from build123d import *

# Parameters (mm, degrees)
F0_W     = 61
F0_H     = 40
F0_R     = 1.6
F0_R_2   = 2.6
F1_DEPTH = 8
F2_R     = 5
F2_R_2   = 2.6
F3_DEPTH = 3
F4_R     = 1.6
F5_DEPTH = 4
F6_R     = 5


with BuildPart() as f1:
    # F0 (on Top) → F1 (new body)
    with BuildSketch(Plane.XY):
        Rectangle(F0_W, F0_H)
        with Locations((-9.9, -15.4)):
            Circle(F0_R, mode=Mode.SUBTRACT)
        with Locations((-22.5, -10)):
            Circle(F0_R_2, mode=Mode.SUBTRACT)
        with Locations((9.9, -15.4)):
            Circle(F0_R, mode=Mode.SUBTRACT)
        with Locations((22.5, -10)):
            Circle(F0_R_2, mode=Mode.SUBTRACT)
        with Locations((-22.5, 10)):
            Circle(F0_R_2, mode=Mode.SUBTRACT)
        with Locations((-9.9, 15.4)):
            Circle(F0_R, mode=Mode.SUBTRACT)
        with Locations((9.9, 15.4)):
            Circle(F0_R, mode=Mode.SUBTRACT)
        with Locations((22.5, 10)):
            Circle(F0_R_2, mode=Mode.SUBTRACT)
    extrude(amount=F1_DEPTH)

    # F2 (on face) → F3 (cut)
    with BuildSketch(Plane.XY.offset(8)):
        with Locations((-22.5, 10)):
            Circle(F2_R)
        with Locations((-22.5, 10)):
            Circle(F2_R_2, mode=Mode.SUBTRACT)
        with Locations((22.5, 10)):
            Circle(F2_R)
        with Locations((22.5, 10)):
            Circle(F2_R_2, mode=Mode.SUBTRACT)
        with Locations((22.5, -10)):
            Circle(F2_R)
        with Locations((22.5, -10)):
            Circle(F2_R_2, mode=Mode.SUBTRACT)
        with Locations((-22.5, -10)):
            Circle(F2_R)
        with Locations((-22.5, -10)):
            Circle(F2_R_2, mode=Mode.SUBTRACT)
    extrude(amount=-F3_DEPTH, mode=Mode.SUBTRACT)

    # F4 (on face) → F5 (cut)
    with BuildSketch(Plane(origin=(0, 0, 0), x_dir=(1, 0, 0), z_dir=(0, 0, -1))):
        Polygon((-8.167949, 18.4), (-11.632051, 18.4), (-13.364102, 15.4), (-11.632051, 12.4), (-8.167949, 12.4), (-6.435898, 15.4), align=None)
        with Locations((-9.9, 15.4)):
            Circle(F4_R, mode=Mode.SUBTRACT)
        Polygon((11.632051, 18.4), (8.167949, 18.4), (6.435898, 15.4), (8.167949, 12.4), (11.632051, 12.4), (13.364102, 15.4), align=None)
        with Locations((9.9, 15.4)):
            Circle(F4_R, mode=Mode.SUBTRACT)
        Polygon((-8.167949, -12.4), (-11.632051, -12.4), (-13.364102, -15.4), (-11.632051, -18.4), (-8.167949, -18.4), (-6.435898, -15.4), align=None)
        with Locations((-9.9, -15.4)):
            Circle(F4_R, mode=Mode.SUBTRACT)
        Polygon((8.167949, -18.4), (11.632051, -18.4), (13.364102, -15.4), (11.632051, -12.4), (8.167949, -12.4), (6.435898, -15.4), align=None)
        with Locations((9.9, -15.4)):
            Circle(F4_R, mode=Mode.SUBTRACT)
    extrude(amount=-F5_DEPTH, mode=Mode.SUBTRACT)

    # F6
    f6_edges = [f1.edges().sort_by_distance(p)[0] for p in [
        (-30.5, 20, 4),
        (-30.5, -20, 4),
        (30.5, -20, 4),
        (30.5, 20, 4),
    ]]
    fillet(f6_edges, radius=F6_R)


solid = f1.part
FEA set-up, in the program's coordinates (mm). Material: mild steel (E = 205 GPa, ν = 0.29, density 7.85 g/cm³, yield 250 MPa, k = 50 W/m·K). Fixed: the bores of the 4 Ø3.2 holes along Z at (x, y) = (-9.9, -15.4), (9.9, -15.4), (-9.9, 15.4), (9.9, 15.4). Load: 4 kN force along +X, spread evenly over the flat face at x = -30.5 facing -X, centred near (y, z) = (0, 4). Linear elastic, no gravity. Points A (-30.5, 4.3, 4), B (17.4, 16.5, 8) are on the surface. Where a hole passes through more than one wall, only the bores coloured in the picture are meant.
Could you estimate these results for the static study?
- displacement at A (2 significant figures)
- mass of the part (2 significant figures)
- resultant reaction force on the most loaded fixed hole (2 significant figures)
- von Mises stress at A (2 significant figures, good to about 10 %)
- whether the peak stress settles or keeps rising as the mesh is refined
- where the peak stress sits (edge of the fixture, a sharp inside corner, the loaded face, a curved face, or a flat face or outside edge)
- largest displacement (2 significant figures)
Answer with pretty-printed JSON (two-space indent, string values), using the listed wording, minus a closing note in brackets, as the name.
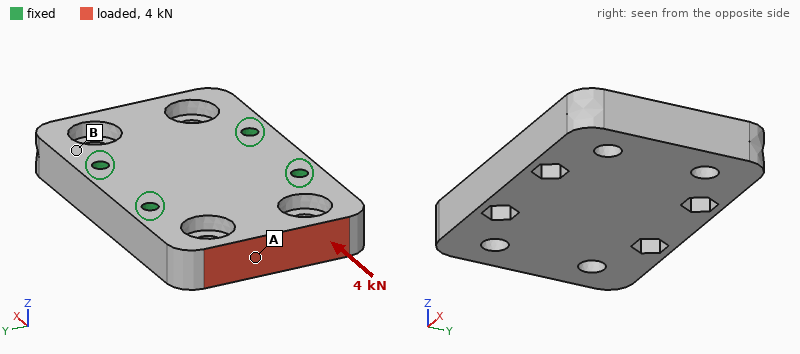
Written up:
{
  "displacement at A": "3.6 µm",
  "mass of the part": "140 g",
  "resultant reaction force on the most loaded fixed hole": "1.4 kN",
  "von Mises stress at A": "17 MPa",
  "whether the peak stress settles or keeps rising as the mesh is refined": "keeps rising",
  "where the peak stress sits": "edge of the fixture",
  "largest displacement": "4.0 µm"
}
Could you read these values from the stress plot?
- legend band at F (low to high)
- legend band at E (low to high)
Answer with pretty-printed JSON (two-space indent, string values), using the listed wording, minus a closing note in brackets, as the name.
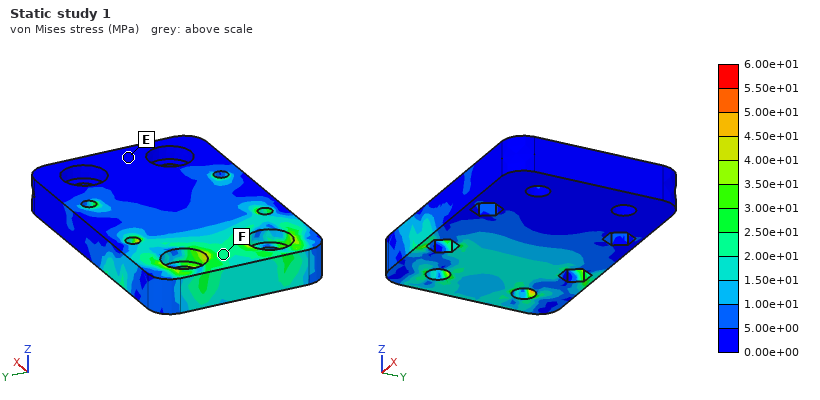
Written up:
{
  "legend band at F": "2.00e+01 to 2.50e+01 MPa",
  "legend band at E": "0.00e+00 to 5.00e+00 MPa"
}
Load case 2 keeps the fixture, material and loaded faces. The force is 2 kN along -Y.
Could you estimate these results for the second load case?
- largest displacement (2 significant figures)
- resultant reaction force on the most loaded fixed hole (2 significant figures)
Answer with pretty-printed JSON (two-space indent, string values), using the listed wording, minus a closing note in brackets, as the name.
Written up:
{
  "largest displacement": "5.5 µm",
  "resultant reaction force on the most loaded fixed hole": "1.4 kN"
}
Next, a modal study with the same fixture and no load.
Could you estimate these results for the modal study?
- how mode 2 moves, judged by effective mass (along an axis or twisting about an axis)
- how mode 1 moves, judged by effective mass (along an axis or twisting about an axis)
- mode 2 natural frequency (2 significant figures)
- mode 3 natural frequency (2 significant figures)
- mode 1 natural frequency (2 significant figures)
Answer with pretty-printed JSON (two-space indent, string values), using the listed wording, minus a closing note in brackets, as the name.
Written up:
{
  "how mode 2 moves, judged by effective mass": "along Z",
  "how mode 1 moves, judged by effective mass": "twisting about Y",
  "mode 2 natural frequency": "9800 Hz",
  "mode 3 natural frequency": "17 kHz",
  "mode 1 natural frequency": "9200 Hz"
}
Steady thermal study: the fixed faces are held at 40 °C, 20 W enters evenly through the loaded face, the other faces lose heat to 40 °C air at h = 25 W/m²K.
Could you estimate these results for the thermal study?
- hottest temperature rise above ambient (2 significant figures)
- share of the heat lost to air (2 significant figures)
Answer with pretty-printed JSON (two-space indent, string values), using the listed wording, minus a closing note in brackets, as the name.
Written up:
{
  "hottest temperature rise above ambient": "42 K",
  "share of the heat lost to air": "7.8 %"
}
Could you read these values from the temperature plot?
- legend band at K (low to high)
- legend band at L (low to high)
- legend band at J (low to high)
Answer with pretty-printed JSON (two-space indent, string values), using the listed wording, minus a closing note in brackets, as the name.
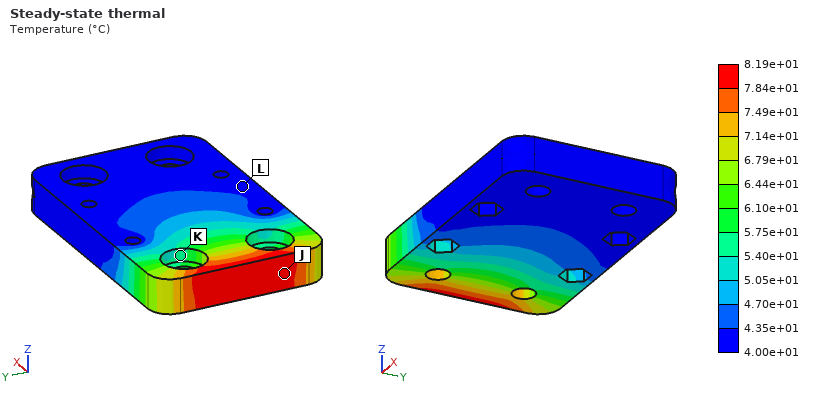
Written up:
{
  "legend band at K": "5.40e+01 to 5.75e+01 °C",
  "legend band at L": "4.00e+01 to 4.35e+01 °C",
  "legend band at J": "7.84e+01 to 8.19e+01 °C"
}
